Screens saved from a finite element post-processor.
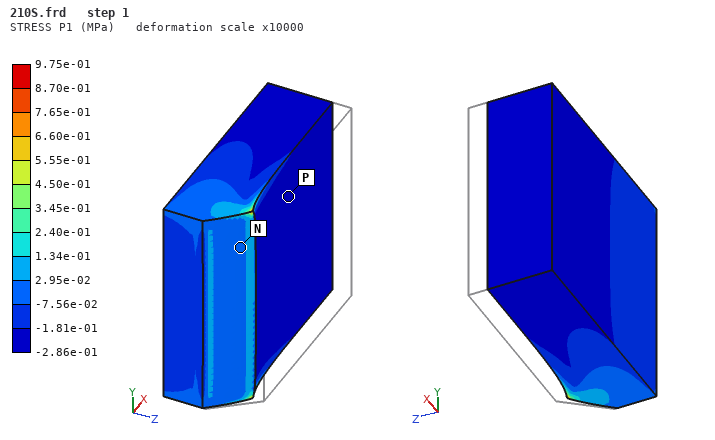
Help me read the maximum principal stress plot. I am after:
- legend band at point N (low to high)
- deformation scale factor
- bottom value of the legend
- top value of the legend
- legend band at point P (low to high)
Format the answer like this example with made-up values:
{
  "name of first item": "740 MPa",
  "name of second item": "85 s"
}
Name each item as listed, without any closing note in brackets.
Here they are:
{
  "legend band at point N": "-7.56e-02 to 2.95e-02 MPa",
  "deformation scale factor": "10000",
  "bottom value of the legend": "-2.86e-01 MPa",
  "top value of the legend": "9.75e-01 MPa",
  "legend band at point P": "-2.86e-01 to -1.81e-01 MPa"
}
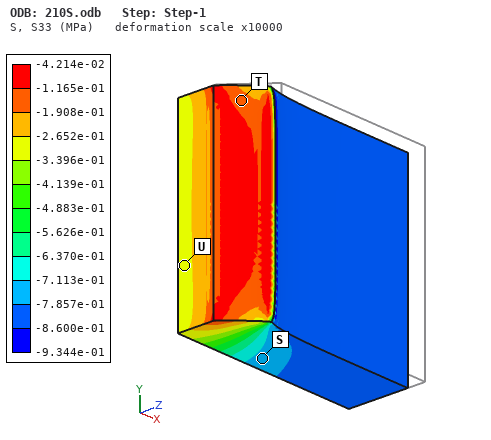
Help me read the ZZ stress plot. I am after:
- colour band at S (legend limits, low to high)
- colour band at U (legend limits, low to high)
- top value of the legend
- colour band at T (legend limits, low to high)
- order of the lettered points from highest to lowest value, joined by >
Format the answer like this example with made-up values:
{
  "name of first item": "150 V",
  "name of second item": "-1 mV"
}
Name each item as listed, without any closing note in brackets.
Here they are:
{
  "colour band at S": "-7.857e-01 to -7.113e-01 MPa",
  "colour band at U": "-3.396e-01 to -2.652e-01 MPa",
  "top value of the legend": "-4.214e-02 MPa",
  "colour band at T": "-1.908e-01 to -1.165e-01 MPa",
  "order of the lettered points from highest to lowest value, joined by >": "T > U > S"
}
